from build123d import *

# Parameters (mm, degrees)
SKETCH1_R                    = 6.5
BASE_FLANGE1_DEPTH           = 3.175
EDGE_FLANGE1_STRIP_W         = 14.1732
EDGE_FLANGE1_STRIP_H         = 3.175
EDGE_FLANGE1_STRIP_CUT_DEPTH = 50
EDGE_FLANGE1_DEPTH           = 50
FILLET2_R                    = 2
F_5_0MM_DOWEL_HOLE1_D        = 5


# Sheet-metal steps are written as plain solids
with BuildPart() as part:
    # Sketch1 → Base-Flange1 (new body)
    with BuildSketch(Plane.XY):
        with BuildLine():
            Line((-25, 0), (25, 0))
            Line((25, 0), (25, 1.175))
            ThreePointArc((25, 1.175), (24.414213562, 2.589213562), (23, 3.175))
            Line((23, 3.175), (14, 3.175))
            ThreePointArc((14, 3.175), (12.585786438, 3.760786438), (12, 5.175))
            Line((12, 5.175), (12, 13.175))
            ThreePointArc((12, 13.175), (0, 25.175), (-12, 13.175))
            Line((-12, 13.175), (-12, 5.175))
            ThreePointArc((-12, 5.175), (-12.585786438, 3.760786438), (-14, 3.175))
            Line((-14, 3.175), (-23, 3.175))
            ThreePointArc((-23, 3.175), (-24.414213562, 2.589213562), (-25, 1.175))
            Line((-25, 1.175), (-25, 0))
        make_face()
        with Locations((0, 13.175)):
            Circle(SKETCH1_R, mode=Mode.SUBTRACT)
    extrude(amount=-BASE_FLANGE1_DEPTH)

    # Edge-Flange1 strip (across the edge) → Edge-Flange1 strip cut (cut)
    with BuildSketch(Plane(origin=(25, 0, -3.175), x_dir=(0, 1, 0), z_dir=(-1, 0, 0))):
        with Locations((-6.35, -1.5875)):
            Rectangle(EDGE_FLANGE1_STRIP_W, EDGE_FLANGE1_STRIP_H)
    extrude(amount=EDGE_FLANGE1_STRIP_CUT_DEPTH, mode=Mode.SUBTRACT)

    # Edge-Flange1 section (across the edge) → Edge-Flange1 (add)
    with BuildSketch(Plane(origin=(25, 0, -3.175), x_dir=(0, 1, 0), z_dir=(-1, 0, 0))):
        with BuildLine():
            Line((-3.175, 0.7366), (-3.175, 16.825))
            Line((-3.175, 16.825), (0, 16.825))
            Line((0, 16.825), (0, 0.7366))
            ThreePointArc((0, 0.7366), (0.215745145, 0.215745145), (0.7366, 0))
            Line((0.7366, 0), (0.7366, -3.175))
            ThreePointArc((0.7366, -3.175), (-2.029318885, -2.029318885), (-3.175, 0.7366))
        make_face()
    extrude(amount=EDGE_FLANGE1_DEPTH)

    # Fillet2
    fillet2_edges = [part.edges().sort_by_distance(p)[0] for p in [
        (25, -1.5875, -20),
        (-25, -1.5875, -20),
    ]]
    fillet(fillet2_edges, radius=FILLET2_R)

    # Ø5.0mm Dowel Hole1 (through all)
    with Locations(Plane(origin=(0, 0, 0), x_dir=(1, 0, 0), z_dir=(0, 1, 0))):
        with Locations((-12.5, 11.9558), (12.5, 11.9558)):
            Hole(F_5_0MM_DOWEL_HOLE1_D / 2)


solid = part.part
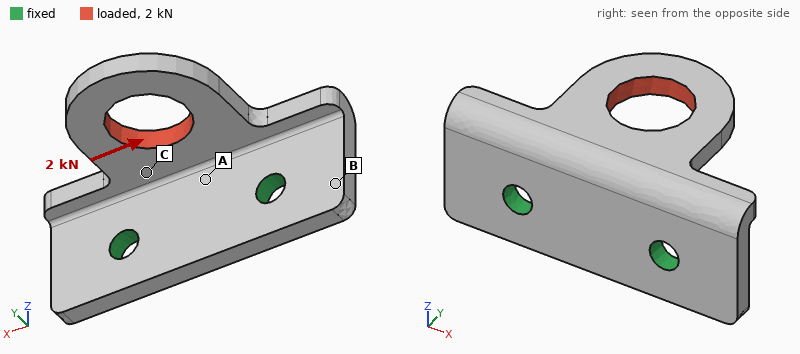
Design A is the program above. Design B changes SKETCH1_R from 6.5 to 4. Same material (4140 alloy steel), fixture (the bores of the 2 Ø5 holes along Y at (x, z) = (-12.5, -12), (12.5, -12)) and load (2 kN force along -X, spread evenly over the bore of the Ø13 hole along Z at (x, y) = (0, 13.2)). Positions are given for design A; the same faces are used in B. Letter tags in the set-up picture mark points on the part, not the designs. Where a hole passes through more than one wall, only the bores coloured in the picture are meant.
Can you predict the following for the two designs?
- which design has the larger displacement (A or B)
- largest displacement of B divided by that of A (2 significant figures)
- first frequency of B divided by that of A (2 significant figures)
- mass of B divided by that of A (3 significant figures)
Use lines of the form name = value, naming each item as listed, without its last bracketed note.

which design has the larger displacement = A
largest displacement of B divided by that of A = 0.85
first frequency of B divided by that of A = 0.96
mass of B divided by that of A = 1.06
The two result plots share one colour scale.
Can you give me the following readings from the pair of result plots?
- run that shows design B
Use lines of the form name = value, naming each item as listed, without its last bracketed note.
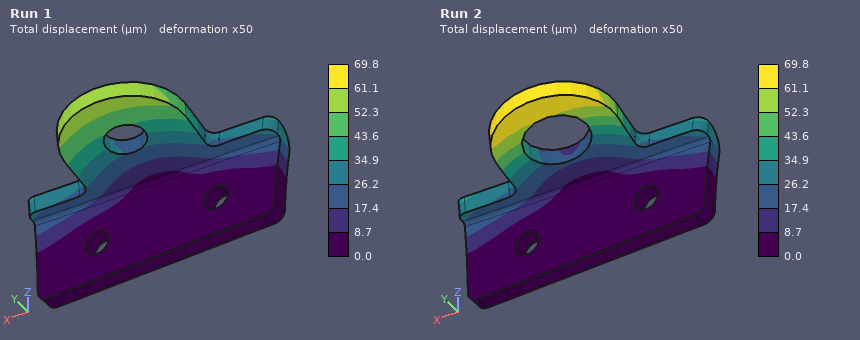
run that shows design B = Run 1
